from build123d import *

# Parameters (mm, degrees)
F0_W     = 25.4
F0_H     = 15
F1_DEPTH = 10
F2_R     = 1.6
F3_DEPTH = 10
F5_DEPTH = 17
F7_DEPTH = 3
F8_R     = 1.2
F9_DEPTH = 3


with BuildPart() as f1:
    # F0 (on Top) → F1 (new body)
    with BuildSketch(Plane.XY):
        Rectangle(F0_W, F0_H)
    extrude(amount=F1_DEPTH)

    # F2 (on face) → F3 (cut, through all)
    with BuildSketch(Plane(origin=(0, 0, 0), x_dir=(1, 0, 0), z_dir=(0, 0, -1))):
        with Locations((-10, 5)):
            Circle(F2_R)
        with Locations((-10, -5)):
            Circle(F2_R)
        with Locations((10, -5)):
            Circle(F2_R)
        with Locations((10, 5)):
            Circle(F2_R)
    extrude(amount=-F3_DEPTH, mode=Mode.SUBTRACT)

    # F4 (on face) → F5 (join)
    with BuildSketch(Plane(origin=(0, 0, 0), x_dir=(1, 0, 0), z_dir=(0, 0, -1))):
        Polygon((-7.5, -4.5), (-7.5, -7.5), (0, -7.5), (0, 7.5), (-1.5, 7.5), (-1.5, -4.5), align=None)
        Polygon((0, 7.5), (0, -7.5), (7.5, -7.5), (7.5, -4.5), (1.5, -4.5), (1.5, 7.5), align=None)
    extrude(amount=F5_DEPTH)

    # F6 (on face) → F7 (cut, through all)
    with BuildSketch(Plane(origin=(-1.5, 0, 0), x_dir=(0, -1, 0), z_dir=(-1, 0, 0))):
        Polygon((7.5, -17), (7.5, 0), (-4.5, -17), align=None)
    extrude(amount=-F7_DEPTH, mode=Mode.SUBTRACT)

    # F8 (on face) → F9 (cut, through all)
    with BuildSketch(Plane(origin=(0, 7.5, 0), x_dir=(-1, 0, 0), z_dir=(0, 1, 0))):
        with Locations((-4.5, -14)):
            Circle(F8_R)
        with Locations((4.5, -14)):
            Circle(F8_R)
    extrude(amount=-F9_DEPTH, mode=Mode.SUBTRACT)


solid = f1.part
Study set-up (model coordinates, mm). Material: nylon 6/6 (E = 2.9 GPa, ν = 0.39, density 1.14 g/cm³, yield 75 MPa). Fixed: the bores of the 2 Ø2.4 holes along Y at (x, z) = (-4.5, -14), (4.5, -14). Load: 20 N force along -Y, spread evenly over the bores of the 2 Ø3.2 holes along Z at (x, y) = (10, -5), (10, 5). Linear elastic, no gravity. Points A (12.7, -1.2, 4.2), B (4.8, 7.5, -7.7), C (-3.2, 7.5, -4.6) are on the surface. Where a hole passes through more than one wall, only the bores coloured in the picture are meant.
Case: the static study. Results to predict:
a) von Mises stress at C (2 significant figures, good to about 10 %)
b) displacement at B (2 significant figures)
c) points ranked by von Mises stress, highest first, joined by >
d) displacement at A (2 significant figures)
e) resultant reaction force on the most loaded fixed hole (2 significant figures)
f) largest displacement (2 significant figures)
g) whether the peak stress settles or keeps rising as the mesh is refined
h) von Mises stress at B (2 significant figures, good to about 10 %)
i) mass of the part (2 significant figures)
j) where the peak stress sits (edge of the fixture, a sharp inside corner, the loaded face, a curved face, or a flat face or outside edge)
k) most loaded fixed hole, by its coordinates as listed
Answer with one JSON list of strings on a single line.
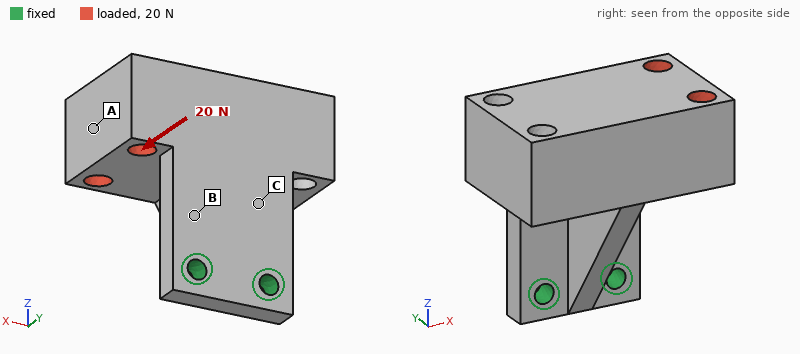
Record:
["3.9 MPa", "0.066 mm", "B > C > A", "0.32 mm", "31 N", "0.42 mm", "keeps rising", "6.5 MPa", "5.2 g", "edge of the fixture", "(4.5, -14)"]
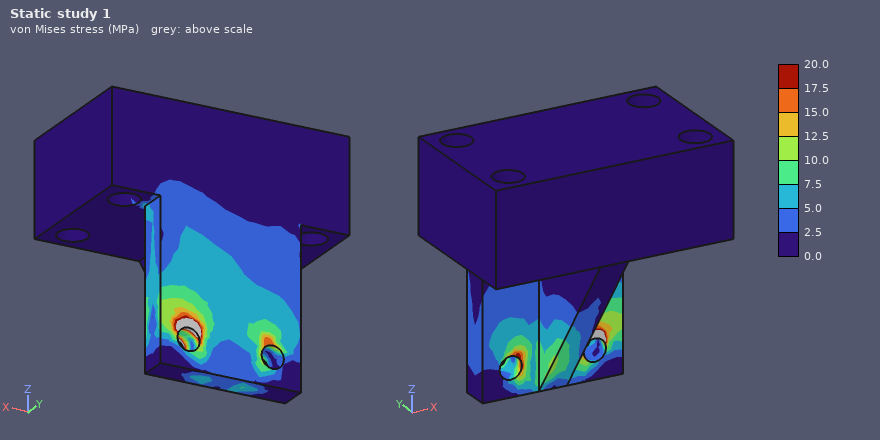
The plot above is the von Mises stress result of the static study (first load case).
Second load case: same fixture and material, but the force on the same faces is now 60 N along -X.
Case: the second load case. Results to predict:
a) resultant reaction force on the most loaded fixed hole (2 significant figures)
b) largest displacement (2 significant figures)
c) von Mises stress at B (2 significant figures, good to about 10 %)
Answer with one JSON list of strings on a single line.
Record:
["120 N", "0.36 mm", "7.2 MPa"]
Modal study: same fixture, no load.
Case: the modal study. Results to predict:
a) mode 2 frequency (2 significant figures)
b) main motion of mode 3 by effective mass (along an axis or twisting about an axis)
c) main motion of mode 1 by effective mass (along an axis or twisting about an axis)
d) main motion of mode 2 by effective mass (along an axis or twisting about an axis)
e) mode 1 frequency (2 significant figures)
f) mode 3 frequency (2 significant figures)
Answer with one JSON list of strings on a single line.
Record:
["1100 Hz", "along X", "along Y", "along X", "720 Hz", "2300 Hz"]
